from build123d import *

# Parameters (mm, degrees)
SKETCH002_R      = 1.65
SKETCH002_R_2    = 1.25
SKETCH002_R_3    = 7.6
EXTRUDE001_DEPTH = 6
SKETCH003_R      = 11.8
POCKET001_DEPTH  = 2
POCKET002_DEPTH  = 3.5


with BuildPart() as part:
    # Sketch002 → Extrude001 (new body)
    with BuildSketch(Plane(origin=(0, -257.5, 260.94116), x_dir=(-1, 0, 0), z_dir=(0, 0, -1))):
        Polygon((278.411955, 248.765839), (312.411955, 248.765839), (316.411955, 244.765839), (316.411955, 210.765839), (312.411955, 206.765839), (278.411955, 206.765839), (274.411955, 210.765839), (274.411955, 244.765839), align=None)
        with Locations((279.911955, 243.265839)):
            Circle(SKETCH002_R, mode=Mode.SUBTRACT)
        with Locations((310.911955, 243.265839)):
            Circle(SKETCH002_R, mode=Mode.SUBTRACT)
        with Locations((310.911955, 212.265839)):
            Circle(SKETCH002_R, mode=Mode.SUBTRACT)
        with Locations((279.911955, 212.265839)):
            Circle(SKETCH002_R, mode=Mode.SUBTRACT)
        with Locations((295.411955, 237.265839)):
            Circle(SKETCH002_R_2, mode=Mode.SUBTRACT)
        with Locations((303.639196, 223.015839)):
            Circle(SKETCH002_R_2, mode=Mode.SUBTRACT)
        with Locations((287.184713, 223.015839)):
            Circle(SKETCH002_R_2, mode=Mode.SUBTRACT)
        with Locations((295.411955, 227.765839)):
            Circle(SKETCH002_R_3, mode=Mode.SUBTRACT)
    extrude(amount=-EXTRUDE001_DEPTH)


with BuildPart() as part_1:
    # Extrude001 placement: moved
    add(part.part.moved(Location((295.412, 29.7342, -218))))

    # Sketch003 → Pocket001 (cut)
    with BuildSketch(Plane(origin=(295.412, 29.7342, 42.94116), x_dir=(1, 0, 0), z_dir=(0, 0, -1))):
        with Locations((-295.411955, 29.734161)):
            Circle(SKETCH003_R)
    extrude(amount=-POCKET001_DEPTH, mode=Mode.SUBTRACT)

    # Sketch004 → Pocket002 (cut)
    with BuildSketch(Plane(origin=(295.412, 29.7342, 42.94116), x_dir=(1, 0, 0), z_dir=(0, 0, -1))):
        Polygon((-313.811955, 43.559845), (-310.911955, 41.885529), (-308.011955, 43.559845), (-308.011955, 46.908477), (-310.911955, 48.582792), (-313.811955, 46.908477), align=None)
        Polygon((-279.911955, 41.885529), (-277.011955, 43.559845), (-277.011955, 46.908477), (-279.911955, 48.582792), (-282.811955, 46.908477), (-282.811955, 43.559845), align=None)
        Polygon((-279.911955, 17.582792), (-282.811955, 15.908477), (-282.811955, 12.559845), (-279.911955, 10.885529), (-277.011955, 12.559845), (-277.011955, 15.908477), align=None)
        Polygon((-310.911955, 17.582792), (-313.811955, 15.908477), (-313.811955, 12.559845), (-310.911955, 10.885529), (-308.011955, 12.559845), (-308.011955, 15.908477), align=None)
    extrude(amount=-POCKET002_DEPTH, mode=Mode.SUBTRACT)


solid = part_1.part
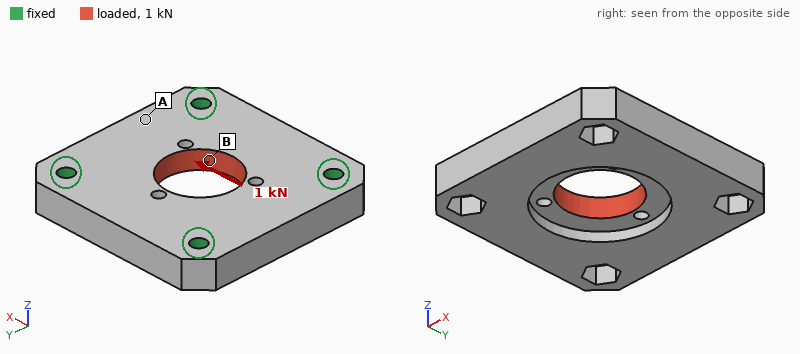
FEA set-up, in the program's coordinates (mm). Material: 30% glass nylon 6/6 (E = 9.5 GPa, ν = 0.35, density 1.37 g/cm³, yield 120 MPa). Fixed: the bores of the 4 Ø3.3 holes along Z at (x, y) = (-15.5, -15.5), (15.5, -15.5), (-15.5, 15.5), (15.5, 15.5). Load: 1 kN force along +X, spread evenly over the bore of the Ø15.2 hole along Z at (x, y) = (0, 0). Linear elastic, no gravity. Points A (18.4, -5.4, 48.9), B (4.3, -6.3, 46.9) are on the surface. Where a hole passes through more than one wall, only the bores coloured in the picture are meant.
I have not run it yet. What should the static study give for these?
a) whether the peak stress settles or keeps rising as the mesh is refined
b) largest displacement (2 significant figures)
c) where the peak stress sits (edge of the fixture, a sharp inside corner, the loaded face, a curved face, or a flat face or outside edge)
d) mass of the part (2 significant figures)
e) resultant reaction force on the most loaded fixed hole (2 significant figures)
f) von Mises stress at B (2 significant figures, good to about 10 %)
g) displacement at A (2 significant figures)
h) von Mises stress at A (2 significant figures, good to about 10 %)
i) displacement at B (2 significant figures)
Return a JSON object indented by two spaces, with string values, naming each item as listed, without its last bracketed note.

{
  "whether the peak stress settles or keeps rising as the mesh is refined": "keeps rising",
  "largest displacement": "18 µm",
  "where the peak stress sits": "edge of the fixture",
  "mass of the part": "11 g",
  "resultant reaction force on the most loaded fixed hole": "260 N",
  "von Mises stress at B": "11 MPa",
  "displacement at A": "11 µm",
  "von Mises stress at A": "2.9 MPa",
  "displacement at B": "13 µm"
}
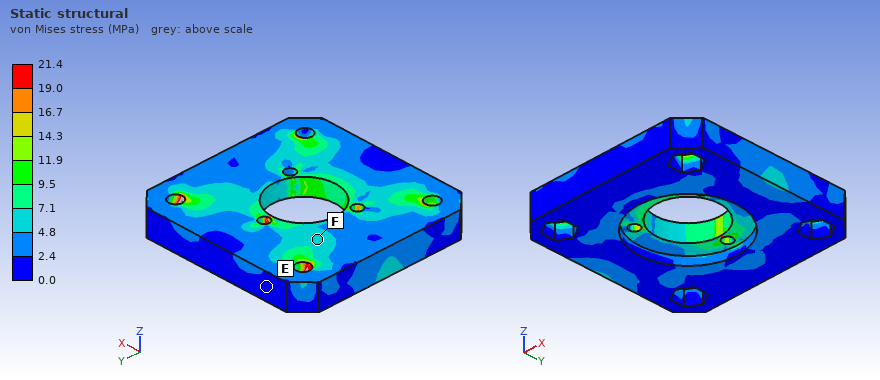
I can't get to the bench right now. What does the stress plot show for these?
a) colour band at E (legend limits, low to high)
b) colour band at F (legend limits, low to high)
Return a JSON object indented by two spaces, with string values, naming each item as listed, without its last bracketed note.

{
  "colour band at E": "0.0 to 2.4 MPa",
  "colour band at F": "4.8 to 7.1 MPa"
}
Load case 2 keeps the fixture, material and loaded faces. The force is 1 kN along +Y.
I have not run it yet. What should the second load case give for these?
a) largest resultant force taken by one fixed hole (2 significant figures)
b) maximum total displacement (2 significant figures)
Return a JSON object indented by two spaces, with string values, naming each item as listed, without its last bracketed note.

{
  "largest resultant force taken by one fixed hole": "260 N",
  "maximum total displacement": "20 µm"
}
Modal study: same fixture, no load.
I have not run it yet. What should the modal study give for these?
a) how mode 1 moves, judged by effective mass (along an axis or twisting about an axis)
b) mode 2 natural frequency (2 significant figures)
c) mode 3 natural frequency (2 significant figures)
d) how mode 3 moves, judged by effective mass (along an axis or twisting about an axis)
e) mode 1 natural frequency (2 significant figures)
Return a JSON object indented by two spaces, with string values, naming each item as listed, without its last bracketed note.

{
  "how mode 1 moves, judged by effective mass": "along Z",
  "mode 2 natural frequency": "10 kHz",
  "mode 3 natural frequency": "11 kHz",
  "how mode 3 moves, judged by effective mass": "twisting about X",
  "mode 1 natural frequency": "8500 Hz"
}
